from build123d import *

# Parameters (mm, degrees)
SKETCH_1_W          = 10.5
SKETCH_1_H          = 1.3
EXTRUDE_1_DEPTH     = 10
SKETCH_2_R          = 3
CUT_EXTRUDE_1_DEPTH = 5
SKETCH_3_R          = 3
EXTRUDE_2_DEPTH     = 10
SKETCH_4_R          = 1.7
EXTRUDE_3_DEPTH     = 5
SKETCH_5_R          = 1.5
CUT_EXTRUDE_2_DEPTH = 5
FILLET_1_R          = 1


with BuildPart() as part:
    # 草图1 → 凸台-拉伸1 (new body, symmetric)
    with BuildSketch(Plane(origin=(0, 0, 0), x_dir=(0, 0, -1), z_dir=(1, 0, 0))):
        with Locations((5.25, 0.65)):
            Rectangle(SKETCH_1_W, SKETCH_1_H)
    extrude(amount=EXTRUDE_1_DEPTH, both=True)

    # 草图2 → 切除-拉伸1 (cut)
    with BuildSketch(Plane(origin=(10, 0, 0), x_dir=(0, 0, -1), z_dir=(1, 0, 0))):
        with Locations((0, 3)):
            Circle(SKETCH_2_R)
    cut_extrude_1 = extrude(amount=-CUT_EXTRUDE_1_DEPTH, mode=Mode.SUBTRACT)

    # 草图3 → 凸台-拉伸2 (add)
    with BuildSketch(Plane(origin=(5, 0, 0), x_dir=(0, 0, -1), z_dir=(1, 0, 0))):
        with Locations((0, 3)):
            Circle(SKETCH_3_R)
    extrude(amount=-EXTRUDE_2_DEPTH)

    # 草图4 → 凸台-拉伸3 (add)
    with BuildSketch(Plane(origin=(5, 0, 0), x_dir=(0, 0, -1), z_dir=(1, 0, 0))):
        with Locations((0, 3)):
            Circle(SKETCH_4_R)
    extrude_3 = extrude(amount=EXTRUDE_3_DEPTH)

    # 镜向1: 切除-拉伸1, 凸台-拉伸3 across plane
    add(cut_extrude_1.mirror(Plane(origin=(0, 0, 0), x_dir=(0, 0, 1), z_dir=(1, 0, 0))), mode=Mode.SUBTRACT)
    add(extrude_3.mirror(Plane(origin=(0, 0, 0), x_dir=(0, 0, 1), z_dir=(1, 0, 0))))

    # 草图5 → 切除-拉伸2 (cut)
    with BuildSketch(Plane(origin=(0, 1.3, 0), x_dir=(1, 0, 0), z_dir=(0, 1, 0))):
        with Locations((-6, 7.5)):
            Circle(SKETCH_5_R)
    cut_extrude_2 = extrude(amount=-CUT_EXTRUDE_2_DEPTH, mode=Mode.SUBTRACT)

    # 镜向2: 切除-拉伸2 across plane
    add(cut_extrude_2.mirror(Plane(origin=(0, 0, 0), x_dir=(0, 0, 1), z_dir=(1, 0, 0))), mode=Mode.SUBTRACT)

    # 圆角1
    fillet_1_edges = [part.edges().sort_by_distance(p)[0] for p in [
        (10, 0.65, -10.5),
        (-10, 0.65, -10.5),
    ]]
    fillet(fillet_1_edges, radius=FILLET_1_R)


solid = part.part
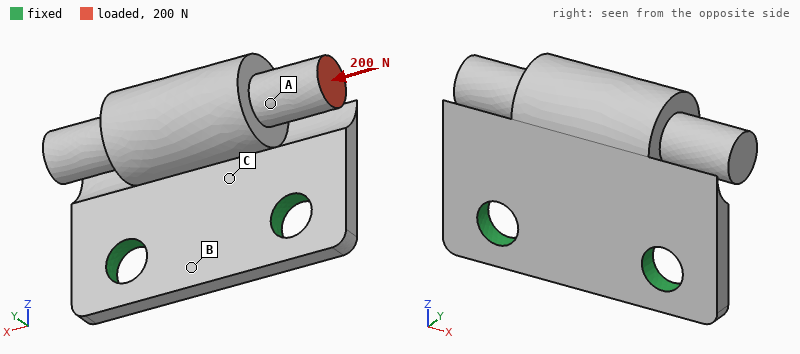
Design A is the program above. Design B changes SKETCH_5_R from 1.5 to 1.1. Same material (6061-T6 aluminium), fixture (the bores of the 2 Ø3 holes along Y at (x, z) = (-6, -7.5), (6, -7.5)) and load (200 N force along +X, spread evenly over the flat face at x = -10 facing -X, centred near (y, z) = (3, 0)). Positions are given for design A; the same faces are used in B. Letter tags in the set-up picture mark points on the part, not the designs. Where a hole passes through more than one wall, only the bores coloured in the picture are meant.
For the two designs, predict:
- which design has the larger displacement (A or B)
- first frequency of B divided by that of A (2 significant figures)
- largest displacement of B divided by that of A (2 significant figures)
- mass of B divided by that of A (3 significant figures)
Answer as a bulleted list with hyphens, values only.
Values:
- B
- 0.92
- 1.2
- 1.01
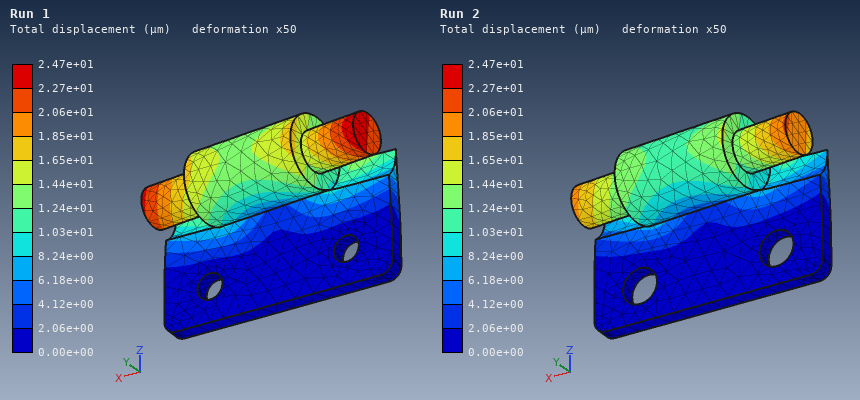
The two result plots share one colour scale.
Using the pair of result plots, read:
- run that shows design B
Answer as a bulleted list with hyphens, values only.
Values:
- Run 1
